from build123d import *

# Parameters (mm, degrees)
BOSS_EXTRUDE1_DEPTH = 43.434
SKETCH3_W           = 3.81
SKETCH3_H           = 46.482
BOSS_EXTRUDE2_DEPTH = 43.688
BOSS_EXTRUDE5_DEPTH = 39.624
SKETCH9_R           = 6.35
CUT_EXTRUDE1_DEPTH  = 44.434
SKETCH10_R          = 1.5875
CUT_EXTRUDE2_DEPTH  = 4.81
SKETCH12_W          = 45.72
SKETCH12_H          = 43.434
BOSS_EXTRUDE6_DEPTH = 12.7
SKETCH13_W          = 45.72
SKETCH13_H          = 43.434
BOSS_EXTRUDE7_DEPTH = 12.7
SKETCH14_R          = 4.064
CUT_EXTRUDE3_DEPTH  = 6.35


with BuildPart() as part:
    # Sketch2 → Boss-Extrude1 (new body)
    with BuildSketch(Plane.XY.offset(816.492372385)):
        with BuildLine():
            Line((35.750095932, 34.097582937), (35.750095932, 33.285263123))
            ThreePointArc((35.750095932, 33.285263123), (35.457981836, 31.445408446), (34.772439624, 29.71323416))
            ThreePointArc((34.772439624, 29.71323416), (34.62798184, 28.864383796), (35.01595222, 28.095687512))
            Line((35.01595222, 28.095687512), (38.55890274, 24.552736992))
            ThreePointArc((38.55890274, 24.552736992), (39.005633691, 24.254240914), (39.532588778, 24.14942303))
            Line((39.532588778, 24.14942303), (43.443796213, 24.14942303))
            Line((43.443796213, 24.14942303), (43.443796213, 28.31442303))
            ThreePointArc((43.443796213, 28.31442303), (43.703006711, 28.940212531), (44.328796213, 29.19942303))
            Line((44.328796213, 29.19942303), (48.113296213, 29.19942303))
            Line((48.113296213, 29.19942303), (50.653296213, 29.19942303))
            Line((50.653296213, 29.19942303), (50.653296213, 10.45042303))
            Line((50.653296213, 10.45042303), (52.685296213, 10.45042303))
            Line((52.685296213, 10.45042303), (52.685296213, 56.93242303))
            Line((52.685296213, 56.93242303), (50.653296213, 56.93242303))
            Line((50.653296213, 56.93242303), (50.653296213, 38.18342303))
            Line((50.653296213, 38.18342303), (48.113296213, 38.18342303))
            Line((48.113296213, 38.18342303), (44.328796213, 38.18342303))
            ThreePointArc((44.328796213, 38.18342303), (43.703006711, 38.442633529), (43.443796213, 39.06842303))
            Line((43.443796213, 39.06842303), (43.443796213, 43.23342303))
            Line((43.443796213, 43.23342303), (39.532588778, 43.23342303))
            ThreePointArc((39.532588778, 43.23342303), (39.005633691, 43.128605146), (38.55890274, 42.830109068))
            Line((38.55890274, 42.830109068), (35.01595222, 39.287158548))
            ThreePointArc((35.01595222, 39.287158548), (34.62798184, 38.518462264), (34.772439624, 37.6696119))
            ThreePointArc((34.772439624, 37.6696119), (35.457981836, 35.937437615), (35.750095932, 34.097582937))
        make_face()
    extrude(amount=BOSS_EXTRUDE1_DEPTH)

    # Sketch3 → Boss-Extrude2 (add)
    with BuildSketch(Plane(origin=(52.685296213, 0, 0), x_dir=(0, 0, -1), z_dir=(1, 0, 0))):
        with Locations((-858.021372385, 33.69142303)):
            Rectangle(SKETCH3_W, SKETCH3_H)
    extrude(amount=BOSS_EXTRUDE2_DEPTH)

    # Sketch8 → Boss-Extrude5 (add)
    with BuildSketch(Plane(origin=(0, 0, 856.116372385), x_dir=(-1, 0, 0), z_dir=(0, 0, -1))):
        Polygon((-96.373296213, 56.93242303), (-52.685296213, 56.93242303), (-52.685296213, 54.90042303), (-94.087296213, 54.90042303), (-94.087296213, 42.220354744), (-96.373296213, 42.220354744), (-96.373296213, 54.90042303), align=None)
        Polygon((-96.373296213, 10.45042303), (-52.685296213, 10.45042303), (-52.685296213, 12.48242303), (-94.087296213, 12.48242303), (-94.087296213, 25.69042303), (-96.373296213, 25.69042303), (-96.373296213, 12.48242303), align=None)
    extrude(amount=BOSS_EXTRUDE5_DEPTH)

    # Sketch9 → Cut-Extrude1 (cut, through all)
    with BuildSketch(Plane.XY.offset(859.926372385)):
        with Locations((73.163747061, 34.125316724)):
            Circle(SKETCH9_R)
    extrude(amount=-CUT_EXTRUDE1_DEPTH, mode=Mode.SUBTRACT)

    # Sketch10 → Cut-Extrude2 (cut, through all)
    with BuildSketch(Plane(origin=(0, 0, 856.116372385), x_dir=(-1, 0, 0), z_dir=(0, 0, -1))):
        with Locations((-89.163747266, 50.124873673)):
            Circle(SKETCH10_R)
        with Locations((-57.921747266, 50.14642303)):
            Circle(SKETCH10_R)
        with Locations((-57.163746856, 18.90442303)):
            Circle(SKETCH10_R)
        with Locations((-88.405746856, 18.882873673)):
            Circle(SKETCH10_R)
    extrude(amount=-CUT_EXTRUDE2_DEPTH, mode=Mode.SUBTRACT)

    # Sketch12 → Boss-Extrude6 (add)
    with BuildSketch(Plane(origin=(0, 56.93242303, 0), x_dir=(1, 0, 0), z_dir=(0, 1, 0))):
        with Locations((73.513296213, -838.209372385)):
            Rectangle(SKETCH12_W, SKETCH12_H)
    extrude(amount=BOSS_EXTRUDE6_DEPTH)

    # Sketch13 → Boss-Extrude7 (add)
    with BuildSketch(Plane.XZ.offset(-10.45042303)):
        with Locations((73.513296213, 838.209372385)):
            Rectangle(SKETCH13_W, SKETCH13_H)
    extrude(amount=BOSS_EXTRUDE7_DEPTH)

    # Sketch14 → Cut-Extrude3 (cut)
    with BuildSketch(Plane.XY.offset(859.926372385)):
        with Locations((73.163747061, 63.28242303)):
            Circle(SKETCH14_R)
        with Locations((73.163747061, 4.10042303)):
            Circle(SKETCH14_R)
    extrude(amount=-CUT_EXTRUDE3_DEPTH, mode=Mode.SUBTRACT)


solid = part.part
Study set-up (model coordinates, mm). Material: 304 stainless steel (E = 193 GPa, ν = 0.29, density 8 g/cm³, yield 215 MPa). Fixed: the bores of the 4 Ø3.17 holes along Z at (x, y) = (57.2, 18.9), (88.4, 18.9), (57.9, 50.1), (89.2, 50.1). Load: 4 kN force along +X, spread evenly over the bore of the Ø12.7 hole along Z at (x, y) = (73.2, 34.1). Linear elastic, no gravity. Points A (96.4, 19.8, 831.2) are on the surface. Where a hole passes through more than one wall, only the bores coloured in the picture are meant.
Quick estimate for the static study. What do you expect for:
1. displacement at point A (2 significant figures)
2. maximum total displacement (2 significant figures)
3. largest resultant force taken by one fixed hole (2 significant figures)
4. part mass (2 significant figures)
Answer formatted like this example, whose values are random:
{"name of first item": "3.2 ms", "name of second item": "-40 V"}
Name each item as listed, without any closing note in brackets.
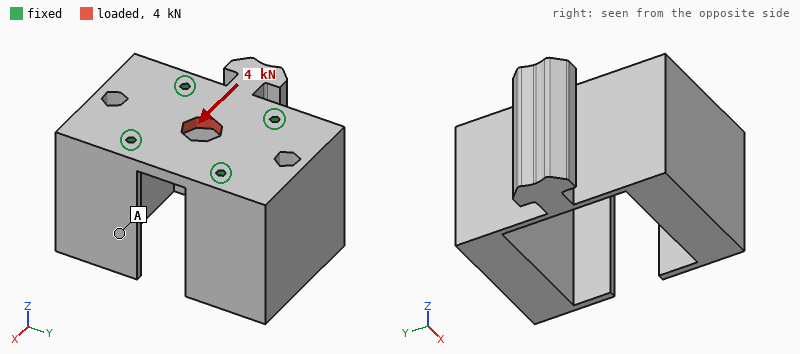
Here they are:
{"displacement at point A": "0.67 µm", "maximum total displacement": "3.0 µm", "largest resultant force taken by one fixed hole": "1.1 kN", "part mass": "640 g"}
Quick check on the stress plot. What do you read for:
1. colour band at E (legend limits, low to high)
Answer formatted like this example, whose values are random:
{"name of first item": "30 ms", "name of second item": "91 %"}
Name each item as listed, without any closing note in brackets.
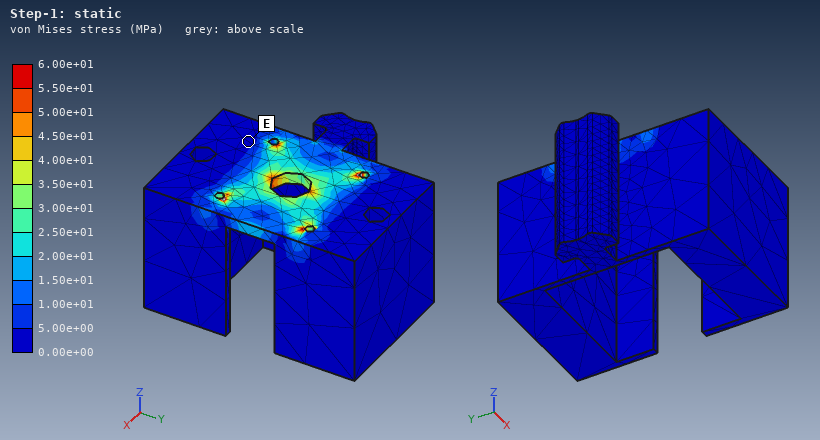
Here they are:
{"colour band at E": "0.00e+00 to 5.00e+00 MPa"}
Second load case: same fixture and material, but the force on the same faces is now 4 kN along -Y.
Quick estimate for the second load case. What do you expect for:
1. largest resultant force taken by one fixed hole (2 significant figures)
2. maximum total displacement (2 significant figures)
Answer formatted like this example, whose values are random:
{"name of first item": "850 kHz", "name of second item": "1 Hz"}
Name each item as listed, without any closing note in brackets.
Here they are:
{"largest resultant force taken by one fixed hole": "1.1 kN", "maximum total displacement": "2.4 µm"}
